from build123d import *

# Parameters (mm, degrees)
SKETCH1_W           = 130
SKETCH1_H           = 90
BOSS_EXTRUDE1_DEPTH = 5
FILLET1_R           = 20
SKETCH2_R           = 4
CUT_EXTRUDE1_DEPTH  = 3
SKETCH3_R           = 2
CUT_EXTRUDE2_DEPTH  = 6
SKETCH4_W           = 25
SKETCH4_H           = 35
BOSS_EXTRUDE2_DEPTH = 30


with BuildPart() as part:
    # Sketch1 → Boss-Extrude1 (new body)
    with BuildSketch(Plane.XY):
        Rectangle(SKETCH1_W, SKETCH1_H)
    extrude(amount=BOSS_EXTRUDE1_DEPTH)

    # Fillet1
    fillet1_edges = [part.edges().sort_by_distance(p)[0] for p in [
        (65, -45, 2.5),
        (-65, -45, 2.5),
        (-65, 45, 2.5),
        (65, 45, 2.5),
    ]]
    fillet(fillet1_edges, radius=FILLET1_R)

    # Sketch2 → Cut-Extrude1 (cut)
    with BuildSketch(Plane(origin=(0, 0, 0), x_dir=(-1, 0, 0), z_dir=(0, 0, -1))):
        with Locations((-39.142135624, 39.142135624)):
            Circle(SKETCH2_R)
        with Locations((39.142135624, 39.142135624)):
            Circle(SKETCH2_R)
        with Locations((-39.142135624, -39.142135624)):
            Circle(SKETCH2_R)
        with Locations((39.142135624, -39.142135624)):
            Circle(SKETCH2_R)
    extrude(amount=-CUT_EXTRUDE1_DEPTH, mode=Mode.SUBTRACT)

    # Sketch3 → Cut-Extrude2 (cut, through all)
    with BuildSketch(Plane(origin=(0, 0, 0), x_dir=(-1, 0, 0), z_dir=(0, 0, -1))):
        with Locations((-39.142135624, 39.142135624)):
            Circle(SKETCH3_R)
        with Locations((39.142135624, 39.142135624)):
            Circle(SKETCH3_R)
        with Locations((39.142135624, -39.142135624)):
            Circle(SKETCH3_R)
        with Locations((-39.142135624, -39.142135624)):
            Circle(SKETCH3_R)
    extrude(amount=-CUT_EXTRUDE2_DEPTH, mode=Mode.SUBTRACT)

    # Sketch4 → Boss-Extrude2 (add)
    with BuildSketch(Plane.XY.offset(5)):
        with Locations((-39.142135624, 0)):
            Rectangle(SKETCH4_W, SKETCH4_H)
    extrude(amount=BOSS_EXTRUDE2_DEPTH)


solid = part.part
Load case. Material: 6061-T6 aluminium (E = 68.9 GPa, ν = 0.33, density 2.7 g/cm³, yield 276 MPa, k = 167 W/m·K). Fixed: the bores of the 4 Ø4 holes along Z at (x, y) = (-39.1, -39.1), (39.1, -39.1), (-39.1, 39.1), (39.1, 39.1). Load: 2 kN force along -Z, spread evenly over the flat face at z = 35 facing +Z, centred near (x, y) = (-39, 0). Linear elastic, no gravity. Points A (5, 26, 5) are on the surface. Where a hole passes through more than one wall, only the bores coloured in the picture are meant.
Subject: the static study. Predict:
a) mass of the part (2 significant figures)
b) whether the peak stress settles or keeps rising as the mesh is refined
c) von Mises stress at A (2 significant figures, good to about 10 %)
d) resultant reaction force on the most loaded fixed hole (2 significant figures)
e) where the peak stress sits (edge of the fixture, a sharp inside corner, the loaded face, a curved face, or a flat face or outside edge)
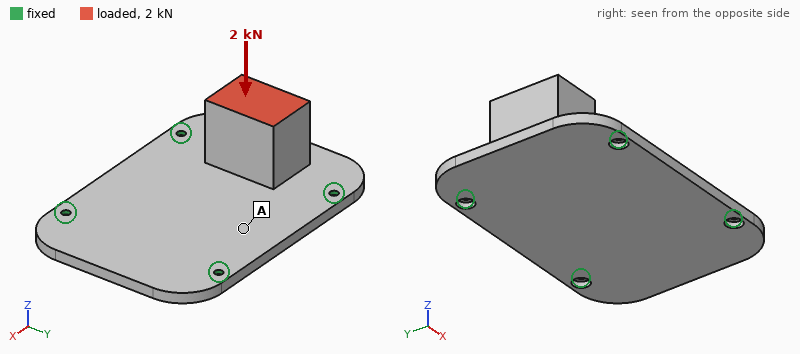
220 g
keeps rising
9.6 MPa
1.4 kN
edge of the fixture
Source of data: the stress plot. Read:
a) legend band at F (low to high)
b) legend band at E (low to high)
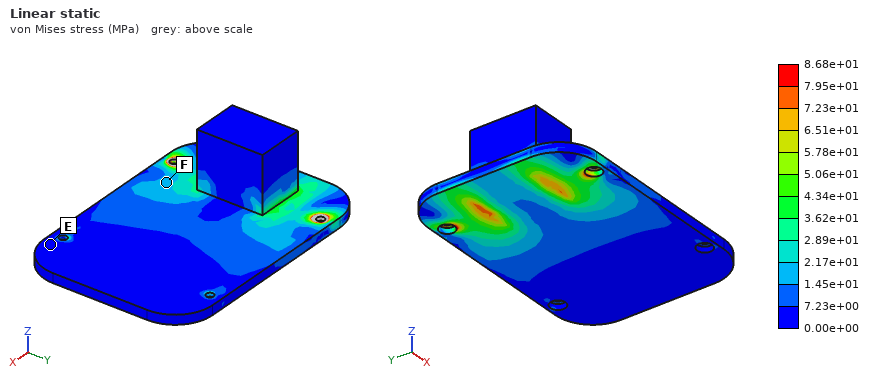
1.45e+01 to 2.17e+01 MPa
0.00e+00 to 7.23e+00 MPa
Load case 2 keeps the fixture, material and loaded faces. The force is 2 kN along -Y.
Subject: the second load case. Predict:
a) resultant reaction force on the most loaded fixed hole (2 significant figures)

1.2 kN
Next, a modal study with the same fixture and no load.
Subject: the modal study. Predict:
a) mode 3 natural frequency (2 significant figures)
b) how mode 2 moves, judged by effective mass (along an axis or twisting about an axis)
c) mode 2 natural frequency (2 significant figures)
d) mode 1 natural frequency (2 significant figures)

2500 Hz
along Z
2000 Hz
1600 Hz
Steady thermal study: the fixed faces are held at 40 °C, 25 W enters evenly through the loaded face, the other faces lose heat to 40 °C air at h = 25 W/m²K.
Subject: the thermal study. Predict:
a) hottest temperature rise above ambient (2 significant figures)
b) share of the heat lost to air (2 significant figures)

16 K
16 %
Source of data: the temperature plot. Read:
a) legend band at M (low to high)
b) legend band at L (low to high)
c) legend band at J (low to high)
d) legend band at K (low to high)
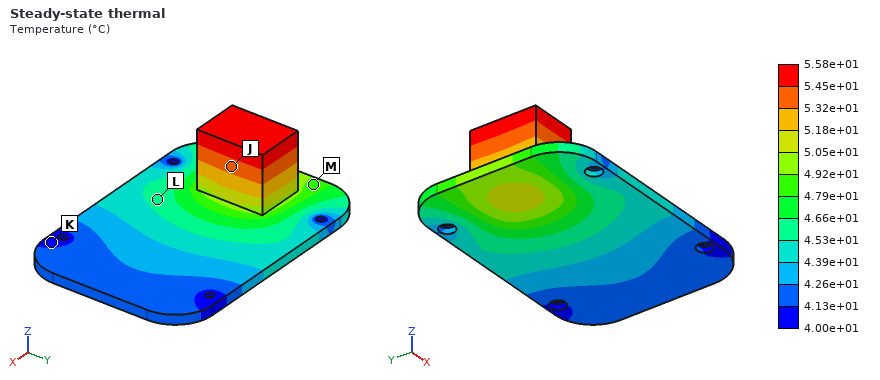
4.79e+01 to 4.92e+01 °C
4.53e+01 to 4.66e+01 °C
5.32e+01 to 5.45e+01 °C
4.00e+01 to 4.13e+01 °C
